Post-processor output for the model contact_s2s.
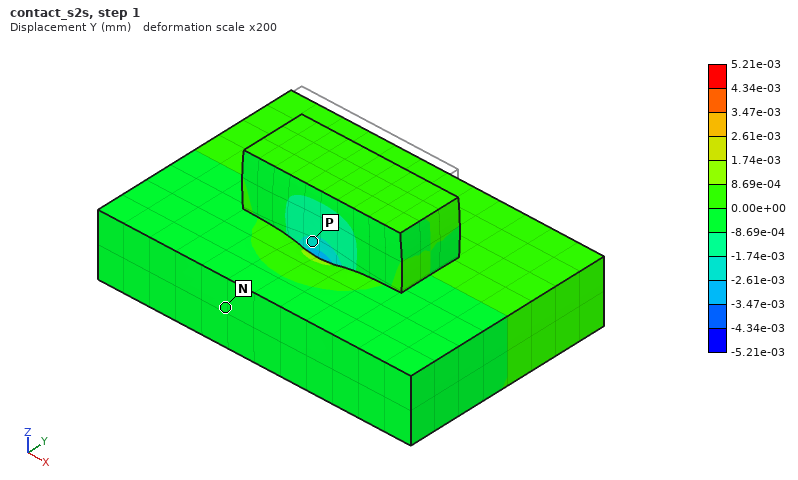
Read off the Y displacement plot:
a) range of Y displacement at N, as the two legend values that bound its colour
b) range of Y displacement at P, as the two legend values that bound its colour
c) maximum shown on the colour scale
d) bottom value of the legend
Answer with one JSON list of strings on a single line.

["-8.69e-04 to 0.00e+00 mm", "-2.61e-03 to -1.74e-03 mm", "5.21e-03 mm", "-5.21e-03 mm"]
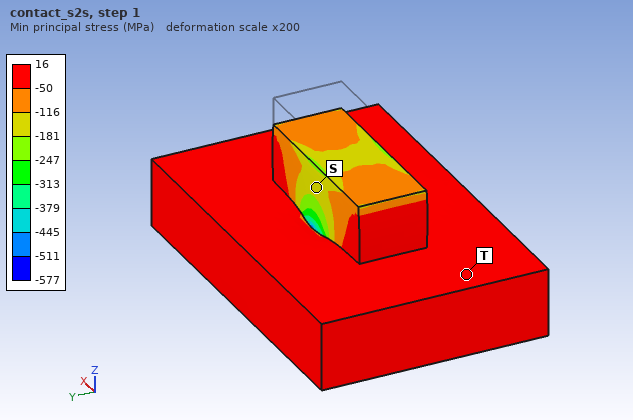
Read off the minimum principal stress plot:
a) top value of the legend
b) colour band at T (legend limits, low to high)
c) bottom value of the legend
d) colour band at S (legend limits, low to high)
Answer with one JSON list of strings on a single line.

["16 MPa", "-50 to 16 MPa", "-577 MPa", "-181 to -116 MPa"]
